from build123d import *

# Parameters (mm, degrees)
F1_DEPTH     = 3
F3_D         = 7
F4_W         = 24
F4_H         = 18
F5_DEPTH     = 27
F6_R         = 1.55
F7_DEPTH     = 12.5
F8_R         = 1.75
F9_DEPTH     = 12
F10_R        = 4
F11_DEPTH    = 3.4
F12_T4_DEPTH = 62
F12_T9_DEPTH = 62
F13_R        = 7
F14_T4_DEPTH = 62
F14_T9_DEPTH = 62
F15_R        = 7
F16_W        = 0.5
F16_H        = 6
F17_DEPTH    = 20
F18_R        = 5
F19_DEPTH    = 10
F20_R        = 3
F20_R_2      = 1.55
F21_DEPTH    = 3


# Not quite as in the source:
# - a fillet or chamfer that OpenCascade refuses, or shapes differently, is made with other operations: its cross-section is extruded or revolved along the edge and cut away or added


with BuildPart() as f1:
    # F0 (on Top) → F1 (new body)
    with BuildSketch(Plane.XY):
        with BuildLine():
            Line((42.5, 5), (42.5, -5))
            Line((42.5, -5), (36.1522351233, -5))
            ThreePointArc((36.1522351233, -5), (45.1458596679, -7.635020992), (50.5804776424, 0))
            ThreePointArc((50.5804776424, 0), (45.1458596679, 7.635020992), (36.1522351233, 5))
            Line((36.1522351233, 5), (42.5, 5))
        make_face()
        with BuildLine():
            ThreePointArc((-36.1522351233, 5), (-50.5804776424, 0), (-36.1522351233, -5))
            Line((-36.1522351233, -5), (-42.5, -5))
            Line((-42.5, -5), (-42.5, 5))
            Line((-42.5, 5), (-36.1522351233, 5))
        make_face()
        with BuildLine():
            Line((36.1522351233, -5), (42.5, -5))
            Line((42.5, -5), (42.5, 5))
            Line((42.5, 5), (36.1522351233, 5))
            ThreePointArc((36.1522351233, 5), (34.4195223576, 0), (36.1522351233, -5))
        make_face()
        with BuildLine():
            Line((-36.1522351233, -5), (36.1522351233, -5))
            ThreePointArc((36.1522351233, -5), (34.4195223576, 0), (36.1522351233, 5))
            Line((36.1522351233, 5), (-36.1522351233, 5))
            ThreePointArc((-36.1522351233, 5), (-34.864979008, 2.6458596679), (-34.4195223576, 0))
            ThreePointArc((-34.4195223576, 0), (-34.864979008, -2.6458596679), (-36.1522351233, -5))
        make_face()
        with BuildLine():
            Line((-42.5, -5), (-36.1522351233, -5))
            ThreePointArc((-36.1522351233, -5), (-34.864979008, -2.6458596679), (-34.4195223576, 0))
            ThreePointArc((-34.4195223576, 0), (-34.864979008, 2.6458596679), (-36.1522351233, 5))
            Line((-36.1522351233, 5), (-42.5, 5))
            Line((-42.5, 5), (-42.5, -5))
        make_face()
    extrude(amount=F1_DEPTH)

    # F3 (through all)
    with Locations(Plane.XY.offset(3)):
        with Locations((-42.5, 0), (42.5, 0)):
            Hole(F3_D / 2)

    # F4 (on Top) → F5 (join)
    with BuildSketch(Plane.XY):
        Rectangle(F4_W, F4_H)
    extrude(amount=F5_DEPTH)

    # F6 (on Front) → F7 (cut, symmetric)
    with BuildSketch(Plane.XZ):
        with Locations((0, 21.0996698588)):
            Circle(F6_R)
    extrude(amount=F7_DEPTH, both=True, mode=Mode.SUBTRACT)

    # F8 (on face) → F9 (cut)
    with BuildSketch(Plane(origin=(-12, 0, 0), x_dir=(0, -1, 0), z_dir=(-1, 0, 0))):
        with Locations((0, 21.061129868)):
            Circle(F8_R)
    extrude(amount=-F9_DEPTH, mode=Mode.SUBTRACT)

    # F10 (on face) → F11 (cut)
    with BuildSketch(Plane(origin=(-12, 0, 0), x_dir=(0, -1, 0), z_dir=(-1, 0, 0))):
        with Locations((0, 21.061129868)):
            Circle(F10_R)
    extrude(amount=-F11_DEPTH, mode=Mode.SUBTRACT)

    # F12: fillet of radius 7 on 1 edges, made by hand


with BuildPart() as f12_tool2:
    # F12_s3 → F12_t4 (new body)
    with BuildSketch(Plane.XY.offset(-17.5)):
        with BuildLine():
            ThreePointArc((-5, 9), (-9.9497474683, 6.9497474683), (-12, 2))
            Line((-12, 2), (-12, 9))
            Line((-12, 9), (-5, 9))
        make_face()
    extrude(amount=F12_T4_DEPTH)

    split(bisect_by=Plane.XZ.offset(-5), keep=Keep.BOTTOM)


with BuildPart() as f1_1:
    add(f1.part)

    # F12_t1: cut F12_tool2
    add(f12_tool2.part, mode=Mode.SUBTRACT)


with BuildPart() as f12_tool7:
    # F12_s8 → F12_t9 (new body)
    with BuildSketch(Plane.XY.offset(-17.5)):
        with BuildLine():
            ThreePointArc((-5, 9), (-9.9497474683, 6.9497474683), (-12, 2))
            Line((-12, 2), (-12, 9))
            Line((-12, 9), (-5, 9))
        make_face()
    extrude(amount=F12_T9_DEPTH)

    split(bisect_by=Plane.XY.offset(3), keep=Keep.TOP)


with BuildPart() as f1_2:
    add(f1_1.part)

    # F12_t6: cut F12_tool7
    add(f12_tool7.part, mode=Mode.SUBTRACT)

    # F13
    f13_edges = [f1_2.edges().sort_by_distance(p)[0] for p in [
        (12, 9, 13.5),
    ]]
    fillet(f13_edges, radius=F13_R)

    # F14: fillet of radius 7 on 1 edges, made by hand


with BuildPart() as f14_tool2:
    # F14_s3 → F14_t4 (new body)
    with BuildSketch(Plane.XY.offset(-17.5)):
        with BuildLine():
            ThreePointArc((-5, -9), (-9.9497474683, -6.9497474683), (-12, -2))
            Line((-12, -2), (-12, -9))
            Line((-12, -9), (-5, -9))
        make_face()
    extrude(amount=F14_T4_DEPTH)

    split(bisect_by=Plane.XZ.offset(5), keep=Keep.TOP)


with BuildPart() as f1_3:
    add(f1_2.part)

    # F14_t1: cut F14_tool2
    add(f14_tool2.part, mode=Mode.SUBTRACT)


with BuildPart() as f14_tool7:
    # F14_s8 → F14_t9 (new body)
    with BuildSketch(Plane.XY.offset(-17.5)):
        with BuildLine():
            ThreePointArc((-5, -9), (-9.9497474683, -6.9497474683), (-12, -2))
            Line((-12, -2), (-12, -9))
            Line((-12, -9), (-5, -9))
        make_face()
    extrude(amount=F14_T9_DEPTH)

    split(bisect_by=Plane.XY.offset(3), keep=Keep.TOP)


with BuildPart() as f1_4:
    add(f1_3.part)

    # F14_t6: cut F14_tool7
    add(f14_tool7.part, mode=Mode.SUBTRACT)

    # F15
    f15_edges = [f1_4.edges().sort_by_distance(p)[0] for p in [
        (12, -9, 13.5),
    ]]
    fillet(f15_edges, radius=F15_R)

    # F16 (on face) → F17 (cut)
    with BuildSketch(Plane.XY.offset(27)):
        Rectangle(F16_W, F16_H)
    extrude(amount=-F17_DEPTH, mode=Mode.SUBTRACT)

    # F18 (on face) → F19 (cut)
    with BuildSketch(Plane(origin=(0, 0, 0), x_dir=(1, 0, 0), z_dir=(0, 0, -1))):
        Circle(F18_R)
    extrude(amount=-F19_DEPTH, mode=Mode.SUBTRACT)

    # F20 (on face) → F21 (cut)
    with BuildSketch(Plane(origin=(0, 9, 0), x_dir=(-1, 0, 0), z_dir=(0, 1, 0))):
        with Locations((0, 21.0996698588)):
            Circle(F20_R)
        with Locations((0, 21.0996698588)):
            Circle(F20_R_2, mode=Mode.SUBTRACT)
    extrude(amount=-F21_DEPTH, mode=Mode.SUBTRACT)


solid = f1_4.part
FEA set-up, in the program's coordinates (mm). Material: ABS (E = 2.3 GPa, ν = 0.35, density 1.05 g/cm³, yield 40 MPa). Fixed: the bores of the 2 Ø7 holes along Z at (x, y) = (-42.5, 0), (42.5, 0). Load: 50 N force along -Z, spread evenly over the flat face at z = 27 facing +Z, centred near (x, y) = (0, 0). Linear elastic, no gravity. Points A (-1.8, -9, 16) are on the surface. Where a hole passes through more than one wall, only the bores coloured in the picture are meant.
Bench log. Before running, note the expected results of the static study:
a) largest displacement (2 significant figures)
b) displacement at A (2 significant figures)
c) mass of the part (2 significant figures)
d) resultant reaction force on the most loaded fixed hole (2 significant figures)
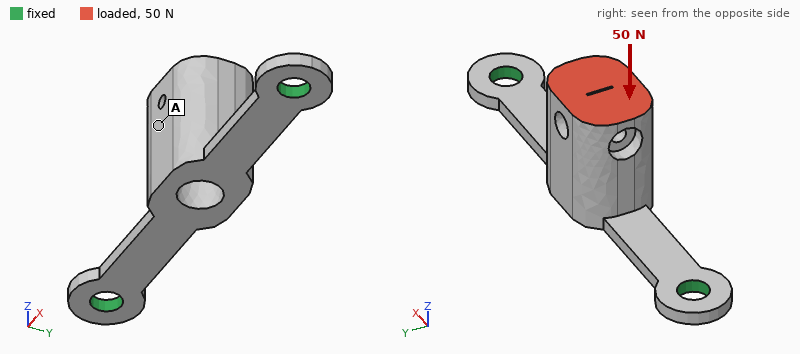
0.95 mm
0.95 mm
12 g
31 N
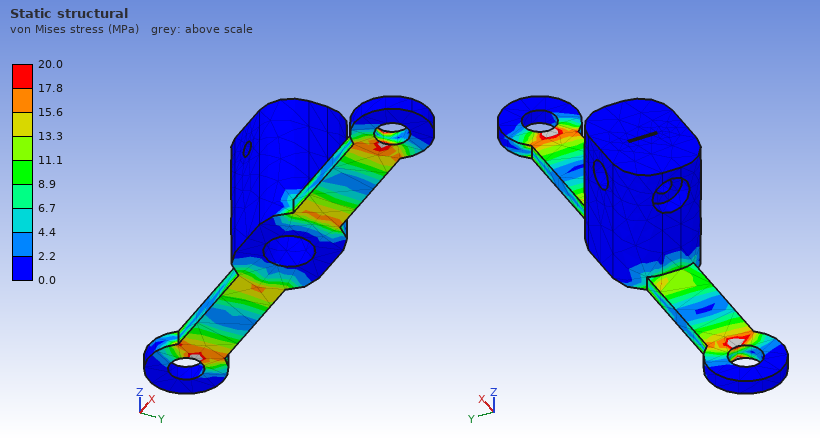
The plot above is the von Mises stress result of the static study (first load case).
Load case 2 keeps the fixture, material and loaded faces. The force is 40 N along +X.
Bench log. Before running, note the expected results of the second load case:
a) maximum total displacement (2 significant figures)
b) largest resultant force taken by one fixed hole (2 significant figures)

0.80 mm
27 N
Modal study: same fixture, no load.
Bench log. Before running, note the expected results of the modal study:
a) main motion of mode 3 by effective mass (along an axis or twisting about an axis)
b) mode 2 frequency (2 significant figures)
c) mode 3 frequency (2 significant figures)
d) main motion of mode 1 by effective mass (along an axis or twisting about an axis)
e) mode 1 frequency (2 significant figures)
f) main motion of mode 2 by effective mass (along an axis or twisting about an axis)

along X
360 Hz
590 Hz
along Y
230 Hz
along Z
